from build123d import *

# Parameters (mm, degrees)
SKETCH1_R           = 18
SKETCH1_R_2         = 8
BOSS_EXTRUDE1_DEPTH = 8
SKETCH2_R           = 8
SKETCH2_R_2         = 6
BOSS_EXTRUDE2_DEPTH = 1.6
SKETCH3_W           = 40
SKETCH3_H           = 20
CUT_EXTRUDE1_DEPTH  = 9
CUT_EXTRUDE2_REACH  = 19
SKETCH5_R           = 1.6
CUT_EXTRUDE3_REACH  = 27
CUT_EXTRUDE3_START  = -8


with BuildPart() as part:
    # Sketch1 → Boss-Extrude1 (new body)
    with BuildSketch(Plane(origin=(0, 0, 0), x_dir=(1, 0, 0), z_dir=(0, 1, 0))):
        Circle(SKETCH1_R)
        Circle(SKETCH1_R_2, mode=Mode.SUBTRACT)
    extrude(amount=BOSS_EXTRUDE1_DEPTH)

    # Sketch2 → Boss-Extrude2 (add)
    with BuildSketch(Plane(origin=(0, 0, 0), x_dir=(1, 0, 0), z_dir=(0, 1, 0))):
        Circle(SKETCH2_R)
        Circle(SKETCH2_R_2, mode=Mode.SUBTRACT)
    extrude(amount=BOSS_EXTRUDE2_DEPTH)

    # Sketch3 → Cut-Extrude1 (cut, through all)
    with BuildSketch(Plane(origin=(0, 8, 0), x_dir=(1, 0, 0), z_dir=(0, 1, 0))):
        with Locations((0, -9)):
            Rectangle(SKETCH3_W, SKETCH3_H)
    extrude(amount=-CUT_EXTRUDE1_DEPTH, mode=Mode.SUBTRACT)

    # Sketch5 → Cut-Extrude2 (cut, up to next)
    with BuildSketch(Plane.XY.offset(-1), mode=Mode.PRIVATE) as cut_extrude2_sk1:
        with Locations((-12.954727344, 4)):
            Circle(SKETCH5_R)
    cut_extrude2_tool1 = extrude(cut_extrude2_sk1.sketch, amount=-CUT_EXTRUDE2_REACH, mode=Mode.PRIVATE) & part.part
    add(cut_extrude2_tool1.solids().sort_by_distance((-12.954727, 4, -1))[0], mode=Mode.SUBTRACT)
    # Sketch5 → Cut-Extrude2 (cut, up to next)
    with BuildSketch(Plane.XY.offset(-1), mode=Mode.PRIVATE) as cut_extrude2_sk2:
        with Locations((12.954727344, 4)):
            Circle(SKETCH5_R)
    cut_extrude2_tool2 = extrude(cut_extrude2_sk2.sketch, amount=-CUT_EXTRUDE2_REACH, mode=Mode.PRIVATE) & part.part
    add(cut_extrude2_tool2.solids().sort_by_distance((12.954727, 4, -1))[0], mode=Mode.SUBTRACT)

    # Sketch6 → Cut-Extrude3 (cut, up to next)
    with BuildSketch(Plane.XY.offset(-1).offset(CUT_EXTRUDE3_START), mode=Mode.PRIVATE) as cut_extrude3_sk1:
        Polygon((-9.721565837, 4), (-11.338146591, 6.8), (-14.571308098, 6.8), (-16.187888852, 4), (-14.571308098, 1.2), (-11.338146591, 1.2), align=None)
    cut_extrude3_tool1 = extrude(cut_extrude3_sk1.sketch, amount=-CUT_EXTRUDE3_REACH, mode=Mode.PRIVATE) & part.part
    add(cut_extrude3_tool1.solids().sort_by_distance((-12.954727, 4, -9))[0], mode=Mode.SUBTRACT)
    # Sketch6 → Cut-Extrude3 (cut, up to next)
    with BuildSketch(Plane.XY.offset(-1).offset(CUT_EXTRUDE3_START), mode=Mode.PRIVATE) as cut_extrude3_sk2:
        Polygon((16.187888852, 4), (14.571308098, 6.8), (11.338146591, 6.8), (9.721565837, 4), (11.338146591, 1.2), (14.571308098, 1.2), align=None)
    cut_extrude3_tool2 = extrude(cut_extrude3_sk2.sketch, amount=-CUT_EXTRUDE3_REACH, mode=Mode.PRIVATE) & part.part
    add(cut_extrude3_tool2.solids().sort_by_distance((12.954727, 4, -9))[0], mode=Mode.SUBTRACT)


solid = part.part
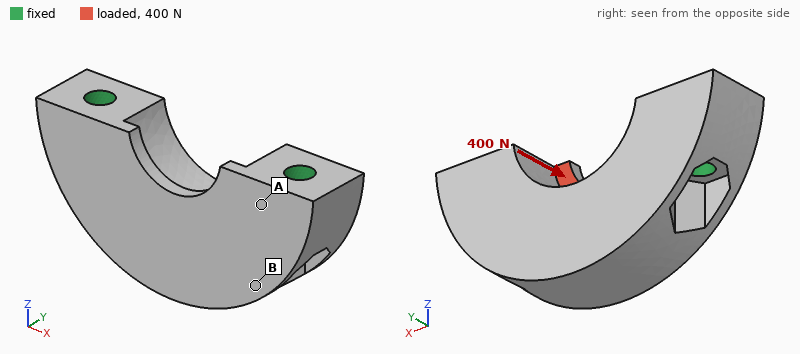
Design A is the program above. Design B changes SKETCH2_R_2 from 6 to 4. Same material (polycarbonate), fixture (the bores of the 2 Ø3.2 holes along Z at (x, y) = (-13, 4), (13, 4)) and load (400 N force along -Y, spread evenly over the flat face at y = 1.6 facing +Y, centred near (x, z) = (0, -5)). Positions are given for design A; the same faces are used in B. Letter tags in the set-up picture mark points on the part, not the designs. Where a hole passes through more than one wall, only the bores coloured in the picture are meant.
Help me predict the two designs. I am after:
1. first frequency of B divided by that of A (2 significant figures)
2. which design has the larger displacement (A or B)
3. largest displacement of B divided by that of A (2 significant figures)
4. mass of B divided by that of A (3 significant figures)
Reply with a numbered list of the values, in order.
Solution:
1. 1.0
2. B
3. 2.3
4. 1.02
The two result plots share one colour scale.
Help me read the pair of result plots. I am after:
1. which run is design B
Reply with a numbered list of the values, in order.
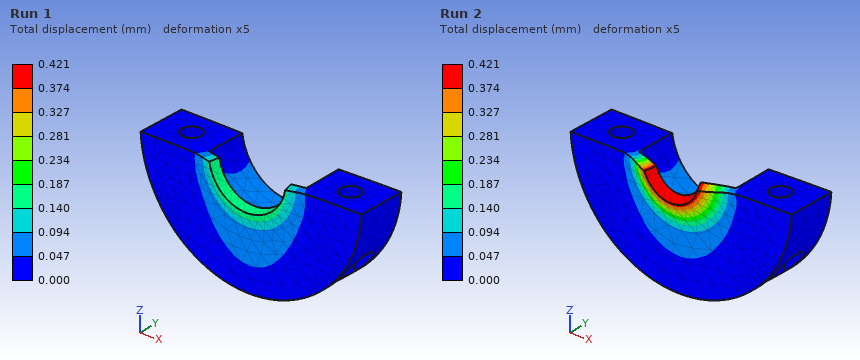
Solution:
1. Run 2
